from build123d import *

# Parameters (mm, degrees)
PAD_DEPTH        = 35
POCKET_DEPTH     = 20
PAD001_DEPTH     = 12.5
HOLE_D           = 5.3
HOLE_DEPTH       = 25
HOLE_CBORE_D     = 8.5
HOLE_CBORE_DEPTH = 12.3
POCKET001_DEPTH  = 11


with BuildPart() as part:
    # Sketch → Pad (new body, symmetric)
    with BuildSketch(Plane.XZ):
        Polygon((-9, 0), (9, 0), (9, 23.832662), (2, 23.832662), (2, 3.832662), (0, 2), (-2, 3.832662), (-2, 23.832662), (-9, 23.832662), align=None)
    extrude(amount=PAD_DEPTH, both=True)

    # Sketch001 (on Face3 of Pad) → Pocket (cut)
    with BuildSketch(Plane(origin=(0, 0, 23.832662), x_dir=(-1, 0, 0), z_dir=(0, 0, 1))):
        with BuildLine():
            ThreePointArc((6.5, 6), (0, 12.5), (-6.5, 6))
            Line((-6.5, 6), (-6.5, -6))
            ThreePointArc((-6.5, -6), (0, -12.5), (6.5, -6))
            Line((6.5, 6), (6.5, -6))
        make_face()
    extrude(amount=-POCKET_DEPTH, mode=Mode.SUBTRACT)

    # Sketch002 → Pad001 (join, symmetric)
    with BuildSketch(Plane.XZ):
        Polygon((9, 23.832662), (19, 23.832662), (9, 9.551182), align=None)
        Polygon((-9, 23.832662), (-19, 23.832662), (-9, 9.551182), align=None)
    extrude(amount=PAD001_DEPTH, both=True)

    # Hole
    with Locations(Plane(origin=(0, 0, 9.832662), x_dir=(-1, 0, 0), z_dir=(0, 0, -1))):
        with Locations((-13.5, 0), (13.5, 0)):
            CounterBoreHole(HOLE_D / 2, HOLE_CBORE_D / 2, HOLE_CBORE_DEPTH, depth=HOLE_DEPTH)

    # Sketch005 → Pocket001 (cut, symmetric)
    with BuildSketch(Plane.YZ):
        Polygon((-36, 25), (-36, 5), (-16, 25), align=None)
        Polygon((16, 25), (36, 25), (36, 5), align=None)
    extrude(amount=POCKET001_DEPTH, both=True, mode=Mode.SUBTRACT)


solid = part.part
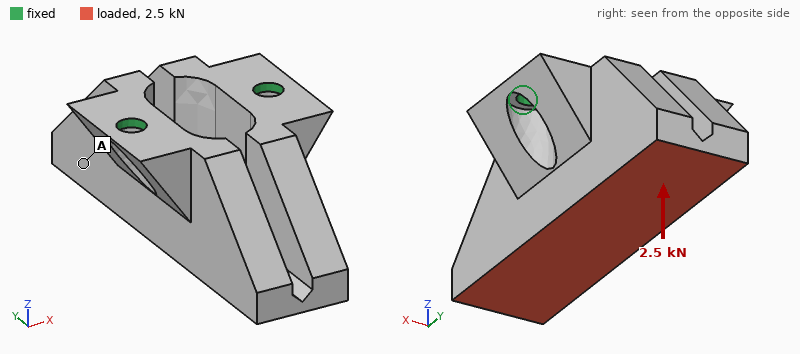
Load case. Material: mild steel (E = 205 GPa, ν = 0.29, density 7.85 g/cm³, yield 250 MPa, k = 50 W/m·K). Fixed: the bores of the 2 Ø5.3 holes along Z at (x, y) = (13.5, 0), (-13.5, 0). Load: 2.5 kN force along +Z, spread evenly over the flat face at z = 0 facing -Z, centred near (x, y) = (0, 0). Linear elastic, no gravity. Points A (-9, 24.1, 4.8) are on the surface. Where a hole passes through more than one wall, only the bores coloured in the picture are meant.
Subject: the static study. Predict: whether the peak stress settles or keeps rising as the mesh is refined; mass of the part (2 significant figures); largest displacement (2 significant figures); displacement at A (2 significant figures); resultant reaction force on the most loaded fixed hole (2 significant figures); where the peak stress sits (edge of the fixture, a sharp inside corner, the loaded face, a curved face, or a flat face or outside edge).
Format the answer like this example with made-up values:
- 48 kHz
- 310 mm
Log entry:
- keeps rising
- 150 g
- 6.8 µm
- 5.5 µm
- 1.3 kN
- edge of the fixture
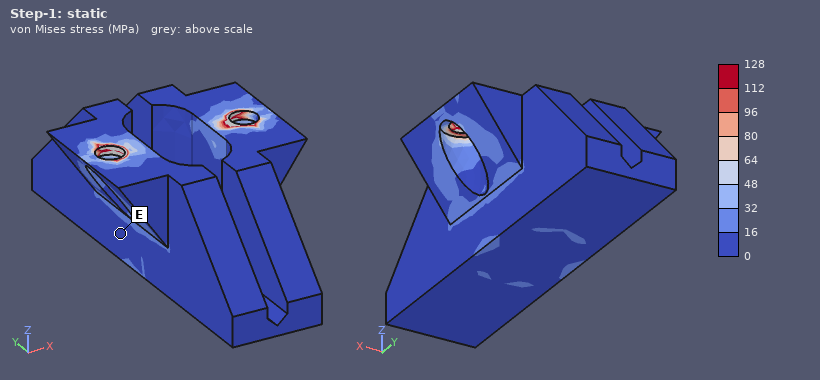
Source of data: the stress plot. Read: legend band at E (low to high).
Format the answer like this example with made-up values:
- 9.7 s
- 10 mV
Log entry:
- 0 to 16 MPa
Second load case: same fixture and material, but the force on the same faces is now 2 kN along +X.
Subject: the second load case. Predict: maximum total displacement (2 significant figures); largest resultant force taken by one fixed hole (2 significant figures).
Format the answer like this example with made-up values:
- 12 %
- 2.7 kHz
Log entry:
- 14 µm
- 2.0 kN
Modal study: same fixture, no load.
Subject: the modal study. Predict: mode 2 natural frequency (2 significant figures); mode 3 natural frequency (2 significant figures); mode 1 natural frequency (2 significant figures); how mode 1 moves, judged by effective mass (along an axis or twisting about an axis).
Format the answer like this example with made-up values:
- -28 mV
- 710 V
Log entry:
- 6900 Hz
- 7000 Hz
- 1500 Hz
- along Y
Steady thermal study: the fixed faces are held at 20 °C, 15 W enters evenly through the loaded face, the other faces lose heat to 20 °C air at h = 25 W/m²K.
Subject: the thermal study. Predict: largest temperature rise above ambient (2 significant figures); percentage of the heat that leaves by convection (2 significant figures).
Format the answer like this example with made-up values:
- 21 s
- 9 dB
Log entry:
- 25 K
- 24 %
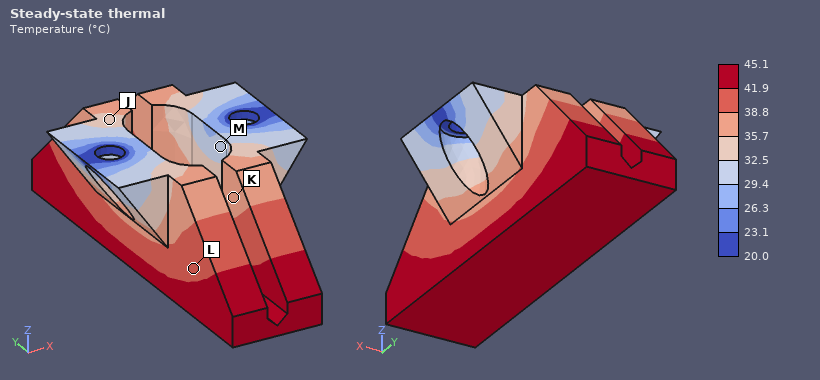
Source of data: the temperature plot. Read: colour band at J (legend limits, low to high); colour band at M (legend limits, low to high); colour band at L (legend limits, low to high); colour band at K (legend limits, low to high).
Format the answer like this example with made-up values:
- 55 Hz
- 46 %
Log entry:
- 32.5 to 35.7 °C
- 29.4 to 32.5 °C
- 38.8 to 41.9 °C
- 35.7 to 38.8 °C
